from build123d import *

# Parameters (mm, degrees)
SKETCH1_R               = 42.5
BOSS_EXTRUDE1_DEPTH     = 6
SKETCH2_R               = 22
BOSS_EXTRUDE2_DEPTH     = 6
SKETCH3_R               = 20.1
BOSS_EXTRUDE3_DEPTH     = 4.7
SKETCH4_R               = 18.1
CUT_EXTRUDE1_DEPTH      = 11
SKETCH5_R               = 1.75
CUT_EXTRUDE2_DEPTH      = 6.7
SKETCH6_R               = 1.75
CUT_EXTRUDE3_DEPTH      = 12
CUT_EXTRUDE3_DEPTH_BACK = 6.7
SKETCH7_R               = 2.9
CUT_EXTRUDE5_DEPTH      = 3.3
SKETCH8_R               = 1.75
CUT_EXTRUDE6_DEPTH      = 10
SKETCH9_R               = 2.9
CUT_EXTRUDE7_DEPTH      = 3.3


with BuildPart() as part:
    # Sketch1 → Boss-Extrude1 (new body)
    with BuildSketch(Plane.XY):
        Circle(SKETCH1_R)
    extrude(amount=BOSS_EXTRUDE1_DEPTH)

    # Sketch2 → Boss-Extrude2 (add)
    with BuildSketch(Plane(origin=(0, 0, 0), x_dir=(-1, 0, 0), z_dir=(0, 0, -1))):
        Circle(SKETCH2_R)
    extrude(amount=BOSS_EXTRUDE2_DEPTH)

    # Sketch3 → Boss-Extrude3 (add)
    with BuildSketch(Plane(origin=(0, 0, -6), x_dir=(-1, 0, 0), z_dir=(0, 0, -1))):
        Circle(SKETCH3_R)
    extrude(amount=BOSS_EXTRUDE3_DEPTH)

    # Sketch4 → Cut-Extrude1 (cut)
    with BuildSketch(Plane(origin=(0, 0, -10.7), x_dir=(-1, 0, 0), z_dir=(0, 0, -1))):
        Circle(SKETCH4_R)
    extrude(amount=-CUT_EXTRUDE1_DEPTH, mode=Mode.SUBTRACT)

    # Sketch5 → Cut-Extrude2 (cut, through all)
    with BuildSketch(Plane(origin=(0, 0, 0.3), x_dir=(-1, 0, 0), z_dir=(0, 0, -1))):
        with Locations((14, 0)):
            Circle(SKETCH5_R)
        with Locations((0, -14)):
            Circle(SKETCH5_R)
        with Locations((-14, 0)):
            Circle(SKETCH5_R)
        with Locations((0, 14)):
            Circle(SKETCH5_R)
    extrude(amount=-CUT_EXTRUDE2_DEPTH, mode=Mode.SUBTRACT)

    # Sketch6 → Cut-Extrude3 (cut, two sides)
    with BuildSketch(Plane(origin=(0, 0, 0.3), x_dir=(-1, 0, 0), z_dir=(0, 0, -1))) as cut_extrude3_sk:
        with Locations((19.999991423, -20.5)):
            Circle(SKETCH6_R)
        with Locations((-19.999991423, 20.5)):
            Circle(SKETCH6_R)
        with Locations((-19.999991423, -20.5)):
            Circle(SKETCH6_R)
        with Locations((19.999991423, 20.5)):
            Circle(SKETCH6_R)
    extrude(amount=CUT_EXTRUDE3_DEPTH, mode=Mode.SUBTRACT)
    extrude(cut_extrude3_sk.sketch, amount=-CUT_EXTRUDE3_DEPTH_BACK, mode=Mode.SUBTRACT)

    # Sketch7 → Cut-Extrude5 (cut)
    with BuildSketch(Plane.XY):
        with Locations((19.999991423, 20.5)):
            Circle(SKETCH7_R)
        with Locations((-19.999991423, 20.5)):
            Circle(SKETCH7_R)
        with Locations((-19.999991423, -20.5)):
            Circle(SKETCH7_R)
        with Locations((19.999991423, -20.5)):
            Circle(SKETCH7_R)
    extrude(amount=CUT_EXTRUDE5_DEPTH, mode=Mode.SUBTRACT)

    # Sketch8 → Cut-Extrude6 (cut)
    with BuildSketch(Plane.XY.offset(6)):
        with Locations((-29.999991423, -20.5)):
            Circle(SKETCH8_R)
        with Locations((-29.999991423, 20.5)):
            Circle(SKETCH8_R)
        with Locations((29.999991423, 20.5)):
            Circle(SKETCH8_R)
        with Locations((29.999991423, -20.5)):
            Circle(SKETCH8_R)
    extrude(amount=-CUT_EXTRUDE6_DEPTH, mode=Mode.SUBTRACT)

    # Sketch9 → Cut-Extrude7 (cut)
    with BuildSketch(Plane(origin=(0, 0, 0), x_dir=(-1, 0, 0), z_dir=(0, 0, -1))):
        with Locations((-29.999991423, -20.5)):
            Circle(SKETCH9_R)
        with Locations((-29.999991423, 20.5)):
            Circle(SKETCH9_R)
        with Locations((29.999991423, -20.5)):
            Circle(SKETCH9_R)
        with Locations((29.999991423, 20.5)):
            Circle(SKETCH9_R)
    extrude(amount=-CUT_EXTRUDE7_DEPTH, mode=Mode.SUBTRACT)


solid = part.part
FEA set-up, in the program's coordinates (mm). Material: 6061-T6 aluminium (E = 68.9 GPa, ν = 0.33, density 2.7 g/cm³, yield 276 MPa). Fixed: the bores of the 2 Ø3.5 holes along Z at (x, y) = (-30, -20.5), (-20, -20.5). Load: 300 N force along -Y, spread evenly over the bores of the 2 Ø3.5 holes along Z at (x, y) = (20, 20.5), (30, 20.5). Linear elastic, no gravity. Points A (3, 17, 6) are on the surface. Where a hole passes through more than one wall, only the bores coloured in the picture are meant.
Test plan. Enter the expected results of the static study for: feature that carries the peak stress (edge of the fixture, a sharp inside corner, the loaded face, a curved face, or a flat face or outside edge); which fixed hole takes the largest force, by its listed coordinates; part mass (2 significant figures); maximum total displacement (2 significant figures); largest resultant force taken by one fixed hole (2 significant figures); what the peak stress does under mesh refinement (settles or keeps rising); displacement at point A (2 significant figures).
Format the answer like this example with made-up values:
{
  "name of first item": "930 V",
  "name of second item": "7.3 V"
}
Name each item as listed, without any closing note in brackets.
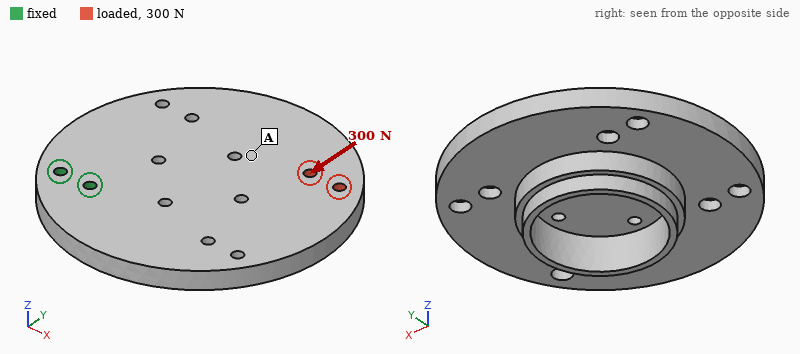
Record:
{
  "feature that carries the peak stress": "edge of the fixture",
  "which fixed hole takes the largest force, by its listed coordinates": "(-20, -20.5)",
  "part mass": "99 g",
  "maximum total displacement": "47 µm",
  "largest resultant force taken by one fixed hole": "1.4 kN",
  "what the peak stress does under mesh refinement": "keeps rising",
  "displacement at point A": "29 µm"
}
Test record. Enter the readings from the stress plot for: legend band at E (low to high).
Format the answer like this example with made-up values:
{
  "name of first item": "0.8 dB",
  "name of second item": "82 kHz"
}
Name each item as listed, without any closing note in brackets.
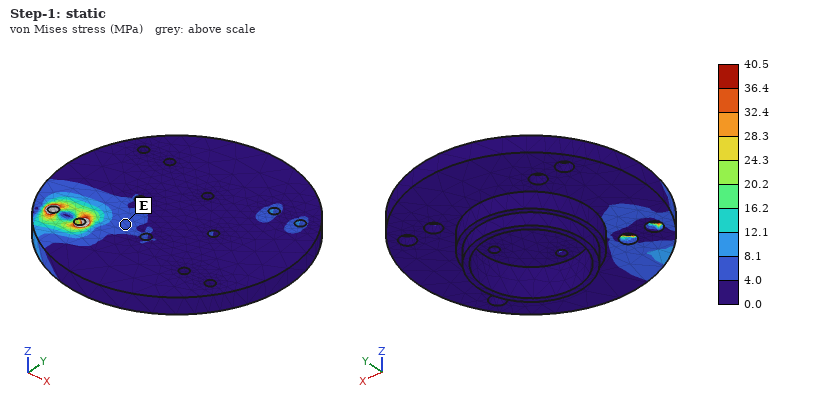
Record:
{
  "legend band at E": "4.0 to 8.1 MPa"
}
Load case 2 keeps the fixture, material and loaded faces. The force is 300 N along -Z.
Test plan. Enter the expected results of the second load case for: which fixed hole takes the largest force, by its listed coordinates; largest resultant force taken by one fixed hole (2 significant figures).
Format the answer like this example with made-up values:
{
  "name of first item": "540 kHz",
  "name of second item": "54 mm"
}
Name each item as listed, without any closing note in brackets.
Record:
{
  "which fixed hole takes the largest force, by its listed coordinates": "(-20, -20.5)",
  "largest resultant force taken by one fixed hole": "1.3 kN"
}
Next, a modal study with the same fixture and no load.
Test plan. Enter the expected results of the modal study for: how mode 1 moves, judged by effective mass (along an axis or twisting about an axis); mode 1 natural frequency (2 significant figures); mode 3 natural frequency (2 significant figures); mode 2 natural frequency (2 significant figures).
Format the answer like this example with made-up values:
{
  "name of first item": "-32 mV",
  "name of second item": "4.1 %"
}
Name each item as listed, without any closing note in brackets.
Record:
{
  "how mode 1 moves, judged by effective mass": "along Z",
  "mode 1 natural frequency": "680 Hz",
  "mode 3 natural frequency": "1800 Hz",
  "mode 2 natural frequency": "1300 Hz"
}
